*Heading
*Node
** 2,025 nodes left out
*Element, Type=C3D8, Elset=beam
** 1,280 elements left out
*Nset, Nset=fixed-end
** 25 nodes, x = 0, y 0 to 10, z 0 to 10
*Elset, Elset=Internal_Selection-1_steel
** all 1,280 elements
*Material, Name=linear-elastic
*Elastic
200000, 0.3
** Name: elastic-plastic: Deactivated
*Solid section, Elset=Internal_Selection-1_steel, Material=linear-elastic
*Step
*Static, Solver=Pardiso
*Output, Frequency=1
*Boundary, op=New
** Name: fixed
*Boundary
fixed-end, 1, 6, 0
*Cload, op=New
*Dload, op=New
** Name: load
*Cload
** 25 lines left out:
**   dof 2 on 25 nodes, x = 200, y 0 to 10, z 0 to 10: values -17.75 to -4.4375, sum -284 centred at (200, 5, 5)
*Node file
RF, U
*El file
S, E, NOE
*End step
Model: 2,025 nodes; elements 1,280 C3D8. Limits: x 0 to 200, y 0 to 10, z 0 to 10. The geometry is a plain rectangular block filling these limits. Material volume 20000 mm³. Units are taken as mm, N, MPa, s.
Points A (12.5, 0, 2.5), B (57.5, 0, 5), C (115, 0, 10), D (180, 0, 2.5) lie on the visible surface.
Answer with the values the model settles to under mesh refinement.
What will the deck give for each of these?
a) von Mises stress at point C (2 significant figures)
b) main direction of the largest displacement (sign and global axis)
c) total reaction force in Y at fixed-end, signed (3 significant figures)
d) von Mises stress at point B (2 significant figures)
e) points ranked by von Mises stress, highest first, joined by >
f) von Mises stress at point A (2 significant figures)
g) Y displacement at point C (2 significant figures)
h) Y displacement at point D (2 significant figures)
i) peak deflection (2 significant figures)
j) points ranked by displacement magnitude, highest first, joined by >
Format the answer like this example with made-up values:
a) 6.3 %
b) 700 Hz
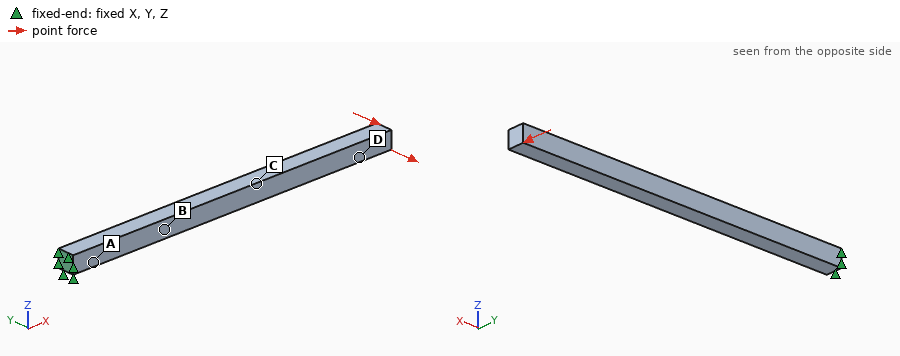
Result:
a) 140 MPa
b) -Y
c) 284 N
d) 240 MPa
e) A > B > C > D
f) 320 MPa
g) -1.8 mm
h) -3.9 mm
i) 4.5 mm
j) D > C > B > A
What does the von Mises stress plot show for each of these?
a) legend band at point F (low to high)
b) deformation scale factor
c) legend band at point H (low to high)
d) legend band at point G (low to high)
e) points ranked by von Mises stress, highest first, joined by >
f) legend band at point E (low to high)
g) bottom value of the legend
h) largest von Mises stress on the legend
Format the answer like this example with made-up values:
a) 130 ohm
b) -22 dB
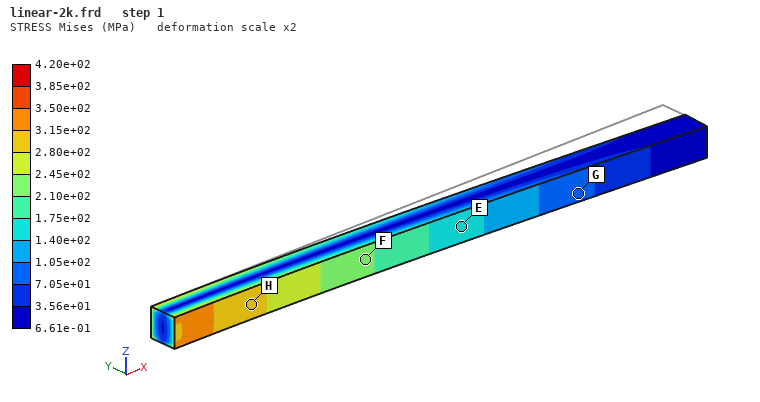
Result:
a) 2.10e+02 to 2.45e+02 MPa
b) 2
c) 2.80e+02 to 3.15e+02 MPa
d) 7.05e+01 to 1.05e+02 MPa
e) H > F > E > G
f) 1.40e+02 to 1.75e+02 MPa
g) 6.61e-01 MPa
h) 4.20e+02 MPa
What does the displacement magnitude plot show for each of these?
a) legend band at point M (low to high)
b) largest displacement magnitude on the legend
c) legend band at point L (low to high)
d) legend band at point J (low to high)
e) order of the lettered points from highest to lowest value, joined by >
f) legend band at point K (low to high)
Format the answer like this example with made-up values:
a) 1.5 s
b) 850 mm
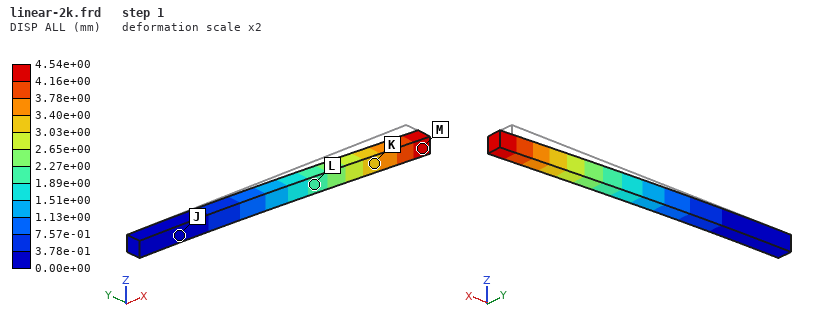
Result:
a) 4.16e+00 to 4.54e+00 mm
b) 4.54e+00 mm
c) 1.89e+00 to 2.27e+00 mm
d) 0.00e+00 to 3.78e-01 mm
e) M > K > L > J
f) 3.03e+00 to 3.40e+00 mm
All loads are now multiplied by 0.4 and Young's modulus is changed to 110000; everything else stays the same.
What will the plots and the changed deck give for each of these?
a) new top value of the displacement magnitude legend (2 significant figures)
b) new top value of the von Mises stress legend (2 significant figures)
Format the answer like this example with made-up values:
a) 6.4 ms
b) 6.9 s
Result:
a) 3.3 mm
b) 170 MPa
